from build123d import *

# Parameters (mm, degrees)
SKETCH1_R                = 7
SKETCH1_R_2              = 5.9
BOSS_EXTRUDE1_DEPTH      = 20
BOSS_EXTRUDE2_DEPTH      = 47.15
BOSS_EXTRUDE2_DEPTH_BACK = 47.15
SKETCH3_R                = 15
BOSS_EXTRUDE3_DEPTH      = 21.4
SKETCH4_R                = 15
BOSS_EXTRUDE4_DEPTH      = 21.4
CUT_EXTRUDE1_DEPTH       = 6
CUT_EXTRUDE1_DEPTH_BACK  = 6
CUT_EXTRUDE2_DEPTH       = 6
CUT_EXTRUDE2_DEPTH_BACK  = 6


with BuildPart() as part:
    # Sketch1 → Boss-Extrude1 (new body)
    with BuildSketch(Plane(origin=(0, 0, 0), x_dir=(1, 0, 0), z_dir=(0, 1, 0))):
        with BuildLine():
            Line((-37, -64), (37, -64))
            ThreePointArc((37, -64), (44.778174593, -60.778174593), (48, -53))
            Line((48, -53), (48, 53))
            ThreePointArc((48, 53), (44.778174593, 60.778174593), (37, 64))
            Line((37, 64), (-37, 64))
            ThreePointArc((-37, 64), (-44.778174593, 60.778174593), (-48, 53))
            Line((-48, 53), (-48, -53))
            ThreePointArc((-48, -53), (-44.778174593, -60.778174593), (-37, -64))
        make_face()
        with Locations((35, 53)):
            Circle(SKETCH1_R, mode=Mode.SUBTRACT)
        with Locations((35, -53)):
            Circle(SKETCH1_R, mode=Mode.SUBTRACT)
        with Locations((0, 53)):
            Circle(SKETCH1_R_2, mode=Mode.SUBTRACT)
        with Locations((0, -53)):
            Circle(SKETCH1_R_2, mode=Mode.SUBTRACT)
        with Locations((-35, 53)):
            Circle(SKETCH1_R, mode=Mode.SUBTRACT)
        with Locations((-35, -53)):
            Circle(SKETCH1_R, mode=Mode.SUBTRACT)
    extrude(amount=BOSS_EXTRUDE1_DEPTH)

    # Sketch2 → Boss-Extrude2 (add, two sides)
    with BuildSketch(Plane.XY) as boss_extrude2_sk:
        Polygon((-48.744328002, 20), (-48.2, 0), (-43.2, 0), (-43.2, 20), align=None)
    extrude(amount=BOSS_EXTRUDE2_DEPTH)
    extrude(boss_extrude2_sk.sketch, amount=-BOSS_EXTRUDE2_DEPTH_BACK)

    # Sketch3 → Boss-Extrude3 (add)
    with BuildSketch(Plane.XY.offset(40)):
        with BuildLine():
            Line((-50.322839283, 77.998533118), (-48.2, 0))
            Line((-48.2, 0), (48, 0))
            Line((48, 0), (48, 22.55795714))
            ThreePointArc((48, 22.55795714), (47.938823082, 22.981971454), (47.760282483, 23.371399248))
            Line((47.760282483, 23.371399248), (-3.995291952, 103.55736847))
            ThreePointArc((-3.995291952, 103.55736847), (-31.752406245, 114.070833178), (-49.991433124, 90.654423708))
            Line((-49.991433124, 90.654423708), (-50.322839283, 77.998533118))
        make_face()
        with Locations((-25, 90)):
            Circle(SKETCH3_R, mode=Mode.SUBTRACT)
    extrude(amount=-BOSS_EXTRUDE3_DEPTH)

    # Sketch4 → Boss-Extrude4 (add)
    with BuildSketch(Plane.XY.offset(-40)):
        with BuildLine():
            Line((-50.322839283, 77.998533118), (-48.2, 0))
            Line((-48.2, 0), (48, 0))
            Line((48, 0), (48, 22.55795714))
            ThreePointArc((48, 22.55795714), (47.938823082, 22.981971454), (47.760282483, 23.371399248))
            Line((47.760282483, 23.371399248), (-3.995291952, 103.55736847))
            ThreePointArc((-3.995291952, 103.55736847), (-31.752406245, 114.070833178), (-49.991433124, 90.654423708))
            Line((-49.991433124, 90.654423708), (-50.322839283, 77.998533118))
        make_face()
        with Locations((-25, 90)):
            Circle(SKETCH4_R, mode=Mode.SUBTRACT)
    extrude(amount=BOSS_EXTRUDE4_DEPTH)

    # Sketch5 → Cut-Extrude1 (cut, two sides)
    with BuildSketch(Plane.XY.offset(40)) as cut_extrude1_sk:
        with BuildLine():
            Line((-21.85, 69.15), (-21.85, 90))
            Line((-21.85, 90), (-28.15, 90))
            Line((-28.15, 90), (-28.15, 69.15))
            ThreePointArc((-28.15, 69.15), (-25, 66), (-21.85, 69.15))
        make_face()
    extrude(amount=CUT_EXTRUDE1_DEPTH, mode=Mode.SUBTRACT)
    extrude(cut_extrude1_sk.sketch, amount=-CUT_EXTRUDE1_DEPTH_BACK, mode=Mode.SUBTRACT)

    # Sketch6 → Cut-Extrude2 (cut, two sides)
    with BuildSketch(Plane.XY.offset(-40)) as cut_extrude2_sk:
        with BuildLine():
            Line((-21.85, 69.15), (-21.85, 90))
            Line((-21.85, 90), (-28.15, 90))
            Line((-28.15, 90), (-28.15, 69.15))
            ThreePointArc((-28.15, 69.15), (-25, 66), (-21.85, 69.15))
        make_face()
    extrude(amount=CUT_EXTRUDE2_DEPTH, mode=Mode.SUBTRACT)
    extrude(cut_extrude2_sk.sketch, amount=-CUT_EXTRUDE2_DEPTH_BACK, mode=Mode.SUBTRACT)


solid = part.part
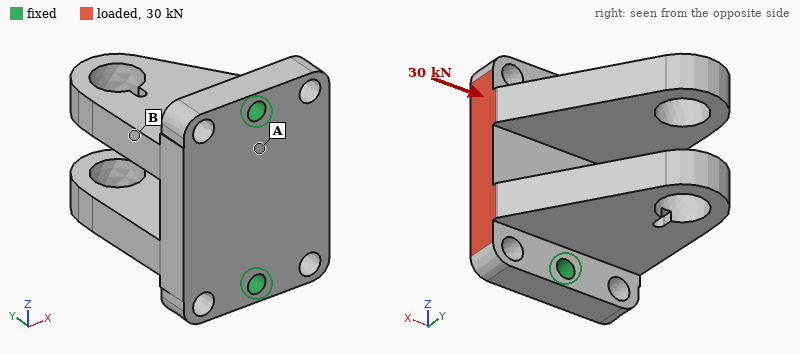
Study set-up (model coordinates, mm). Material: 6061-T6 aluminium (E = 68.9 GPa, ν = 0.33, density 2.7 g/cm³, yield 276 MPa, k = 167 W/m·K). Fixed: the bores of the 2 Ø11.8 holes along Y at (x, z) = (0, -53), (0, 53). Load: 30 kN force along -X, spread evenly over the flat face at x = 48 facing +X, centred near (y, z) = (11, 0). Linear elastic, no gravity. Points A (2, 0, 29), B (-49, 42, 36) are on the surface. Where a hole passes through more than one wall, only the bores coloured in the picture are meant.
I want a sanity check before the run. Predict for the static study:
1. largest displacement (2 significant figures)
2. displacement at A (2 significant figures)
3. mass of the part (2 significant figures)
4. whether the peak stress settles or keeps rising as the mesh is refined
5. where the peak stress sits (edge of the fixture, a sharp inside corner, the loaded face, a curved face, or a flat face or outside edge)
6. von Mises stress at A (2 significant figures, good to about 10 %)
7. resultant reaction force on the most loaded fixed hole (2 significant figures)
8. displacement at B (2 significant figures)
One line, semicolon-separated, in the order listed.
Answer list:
20 µm; 9.6 µm; 1.3 kg; keeps rising; edge of the fixture; 11 MPa; 15 kN; 12 µm
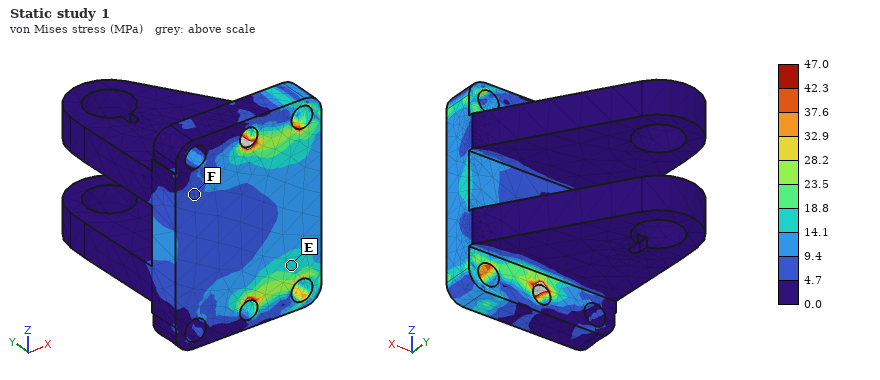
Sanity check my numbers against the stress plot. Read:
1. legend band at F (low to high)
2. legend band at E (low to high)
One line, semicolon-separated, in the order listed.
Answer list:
4.7 to 9.4 MPa; 14.1 to 18.8 MPa
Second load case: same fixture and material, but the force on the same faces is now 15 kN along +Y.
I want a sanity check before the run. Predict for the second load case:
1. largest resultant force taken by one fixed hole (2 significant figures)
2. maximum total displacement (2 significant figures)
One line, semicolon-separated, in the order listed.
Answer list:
7.7 kN; 0.22 mm
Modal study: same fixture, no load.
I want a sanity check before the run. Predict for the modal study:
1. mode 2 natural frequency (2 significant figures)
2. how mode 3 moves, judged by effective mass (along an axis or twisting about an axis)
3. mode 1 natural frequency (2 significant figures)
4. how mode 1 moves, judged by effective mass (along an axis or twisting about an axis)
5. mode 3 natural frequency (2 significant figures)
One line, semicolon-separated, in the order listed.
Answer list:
1900 Hz; along Z; 1800 Hz; along X; 2400 Hz
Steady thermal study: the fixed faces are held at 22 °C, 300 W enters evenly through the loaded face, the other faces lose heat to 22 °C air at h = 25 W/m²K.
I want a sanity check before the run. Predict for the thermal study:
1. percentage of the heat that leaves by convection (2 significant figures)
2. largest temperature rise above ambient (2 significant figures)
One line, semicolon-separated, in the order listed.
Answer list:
8.2 %; 42 K
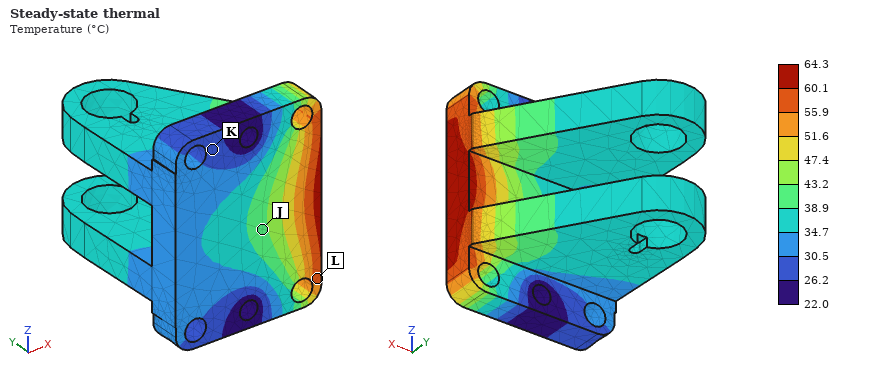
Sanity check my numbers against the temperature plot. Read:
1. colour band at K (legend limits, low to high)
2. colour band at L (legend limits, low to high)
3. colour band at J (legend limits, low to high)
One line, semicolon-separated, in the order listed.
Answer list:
26.2 to 30.5 °C; 55.9 to 60.1 °C; 38.9 to 43.2 °C
